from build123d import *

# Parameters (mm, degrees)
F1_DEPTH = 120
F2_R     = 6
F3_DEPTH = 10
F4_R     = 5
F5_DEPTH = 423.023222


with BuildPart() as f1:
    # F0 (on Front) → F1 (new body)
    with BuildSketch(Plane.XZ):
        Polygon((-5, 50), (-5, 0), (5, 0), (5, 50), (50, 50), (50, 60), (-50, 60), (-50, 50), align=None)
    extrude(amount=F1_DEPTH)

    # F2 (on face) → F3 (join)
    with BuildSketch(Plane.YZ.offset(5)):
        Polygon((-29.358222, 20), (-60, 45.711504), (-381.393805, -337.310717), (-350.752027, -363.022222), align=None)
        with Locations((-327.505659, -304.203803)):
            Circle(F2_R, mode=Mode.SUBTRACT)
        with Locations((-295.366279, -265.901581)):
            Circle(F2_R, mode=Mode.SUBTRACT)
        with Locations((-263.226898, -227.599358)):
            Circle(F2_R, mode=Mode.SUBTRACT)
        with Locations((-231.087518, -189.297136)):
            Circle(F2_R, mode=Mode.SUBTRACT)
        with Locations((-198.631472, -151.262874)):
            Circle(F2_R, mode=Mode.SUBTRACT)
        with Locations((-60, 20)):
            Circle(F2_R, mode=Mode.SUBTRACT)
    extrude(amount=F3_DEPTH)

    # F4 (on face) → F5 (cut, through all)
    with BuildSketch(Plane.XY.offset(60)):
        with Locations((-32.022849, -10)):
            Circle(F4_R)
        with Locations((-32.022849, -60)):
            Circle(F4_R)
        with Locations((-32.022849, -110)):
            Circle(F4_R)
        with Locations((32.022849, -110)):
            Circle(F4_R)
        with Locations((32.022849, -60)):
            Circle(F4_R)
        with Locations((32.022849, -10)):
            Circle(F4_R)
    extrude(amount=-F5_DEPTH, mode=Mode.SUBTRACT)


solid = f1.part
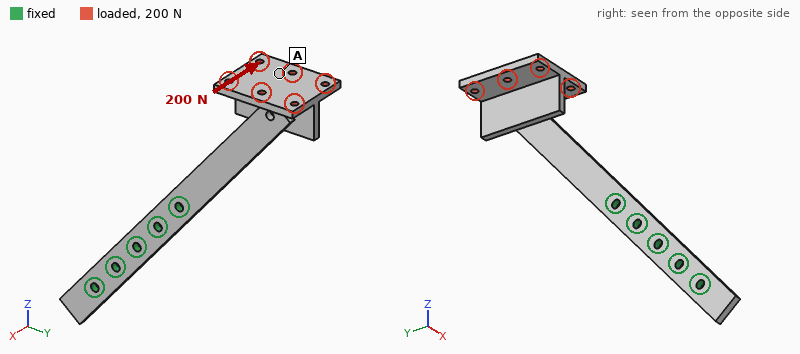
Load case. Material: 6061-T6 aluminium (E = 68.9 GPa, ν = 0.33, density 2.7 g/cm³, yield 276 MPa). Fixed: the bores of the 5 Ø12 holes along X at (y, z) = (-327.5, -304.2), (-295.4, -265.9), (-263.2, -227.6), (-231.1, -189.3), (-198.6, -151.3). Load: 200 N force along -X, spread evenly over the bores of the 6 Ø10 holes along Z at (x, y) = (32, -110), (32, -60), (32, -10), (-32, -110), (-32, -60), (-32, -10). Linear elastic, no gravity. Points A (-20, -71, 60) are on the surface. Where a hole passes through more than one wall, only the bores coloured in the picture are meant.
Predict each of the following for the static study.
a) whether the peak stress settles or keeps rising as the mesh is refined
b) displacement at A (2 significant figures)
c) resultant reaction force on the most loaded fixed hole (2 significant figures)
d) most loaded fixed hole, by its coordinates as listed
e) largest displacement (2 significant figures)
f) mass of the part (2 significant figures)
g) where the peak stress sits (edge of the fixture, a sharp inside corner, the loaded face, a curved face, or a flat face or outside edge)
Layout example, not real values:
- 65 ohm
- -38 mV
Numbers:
- keeps rising
- 4.3 mm
- 290 N
- (-198.6, -151.3)
- 5.4 mm
- 990 g
- edge of the fixture
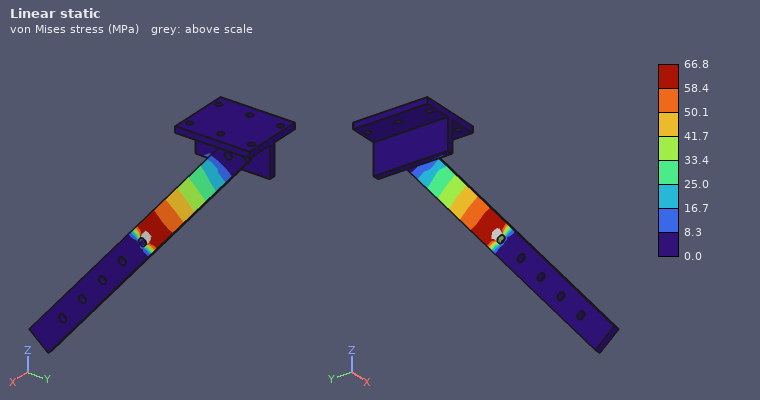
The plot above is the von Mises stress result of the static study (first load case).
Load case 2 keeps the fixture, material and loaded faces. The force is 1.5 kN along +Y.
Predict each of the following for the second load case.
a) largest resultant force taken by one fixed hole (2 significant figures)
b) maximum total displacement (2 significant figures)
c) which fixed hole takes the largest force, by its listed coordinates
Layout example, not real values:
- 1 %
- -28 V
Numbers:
- 4.4 kN
- 3.4 mm
- (-198.6, -151.3)
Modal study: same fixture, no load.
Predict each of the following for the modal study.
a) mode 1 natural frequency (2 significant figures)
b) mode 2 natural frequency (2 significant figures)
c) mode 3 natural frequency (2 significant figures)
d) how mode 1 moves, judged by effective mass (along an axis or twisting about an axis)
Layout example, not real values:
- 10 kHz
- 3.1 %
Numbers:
- 49 Hz
- 170 Hz
- 240 Hz
- along X
